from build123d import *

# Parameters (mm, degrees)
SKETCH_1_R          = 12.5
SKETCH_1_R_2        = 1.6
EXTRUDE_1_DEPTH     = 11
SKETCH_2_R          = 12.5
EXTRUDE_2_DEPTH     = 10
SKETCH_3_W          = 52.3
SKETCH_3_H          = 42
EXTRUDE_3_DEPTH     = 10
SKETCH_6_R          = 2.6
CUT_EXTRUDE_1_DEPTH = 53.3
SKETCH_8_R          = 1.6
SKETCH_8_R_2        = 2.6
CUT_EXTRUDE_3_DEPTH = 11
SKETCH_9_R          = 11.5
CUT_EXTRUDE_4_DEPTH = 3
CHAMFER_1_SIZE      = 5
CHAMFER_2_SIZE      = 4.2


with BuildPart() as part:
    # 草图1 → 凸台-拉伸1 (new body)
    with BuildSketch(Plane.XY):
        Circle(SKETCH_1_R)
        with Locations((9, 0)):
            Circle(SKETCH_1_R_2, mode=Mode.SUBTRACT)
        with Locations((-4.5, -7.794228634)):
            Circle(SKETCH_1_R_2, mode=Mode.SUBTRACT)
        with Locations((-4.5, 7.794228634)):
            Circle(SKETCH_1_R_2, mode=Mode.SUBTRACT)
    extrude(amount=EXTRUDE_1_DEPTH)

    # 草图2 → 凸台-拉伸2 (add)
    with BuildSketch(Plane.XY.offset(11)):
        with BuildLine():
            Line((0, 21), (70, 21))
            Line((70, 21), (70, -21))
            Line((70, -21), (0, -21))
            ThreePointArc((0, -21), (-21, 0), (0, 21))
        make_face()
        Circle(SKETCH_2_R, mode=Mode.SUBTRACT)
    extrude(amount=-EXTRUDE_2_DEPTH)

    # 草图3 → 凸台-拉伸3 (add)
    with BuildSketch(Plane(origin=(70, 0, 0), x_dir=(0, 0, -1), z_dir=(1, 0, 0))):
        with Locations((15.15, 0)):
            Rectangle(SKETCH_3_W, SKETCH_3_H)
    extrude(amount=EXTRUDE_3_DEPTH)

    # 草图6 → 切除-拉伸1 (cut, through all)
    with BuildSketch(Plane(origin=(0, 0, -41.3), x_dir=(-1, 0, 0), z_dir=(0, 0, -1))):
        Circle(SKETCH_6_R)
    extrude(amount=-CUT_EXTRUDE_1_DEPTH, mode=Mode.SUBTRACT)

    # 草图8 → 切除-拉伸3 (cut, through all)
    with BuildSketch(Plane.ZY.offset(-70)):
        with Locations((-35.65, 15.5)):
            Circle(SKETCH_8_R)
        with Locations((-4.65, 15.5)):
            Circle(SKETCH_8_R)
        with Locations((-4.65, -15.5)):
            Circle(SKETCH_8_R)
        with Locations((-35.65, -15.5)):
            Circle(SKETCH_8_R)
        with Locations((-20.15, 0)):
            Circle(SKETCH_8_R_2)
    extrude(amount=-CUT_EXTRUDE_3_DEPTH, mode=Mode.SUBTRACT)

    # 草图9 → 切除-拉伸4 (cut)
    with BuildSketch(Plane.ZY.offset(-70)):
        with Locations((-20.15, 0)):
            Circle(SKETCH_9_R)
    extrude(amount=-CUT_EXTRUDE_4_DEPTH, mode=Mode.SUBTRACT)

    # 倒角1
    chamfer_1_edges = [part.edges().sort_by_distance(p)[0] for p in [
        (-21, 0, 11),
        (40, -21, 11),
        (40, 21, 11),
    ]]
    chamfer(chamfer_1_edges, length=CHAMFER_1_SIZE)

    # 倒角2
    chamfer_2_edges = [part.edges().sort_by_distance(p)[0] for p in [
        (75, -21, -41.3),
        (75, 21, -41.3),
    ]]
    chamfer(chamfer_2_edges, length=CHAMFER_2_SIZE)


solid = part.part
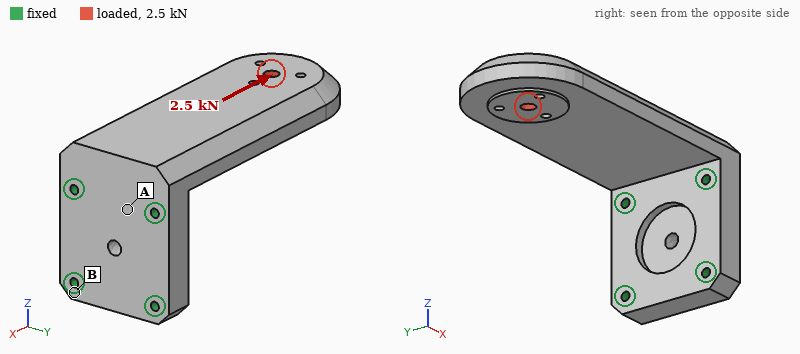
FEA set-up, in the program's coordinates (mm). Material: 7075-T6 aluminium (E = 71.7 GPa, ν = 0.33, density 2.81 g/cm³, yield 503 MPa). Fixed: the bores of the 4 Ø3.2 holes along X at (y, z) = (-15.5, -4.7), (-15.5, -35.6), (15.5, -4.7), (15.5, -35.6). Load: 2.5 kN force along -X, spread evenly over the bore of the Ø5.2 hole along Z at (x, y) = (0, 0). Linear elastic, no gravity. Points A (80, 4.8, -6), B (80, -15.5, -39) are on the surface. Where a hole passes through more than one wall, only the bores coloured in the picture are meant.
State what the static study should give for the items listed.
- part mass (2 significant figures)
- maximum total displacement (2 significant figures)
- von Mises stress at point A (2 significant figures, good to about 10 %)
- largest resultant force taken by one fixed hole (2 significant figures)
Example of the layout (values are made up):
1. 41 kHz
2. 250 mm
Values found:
1. 150 g
2. 76 µm
3. 13 MPa
4. 1.4 kN
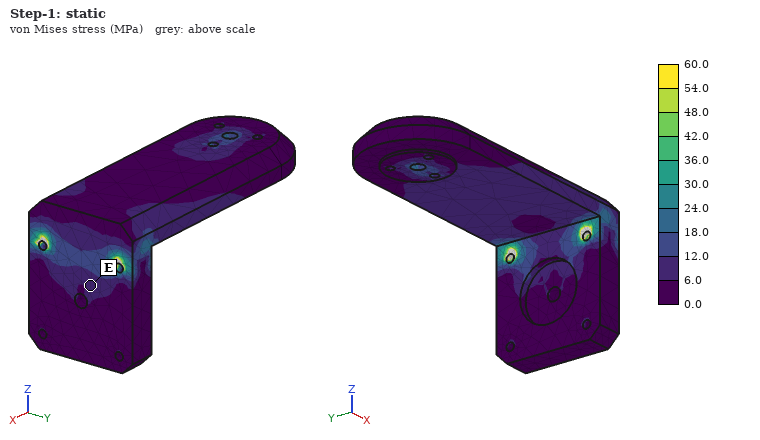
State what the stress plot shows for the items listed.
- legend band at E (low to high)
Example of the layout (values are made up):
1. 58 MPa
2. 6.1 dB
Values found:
1. 6.0 to 12.0 MPa
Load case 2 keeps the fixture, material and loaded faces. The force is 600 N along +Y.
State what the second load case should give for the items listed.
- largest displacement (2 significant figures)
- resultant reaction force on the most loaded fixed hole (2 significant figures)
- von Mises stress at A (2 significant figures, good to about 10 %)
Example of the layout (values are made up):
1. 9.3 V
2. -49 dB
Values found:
1. 73 µm
2. 1.4 kN
3. 7.6 MPa
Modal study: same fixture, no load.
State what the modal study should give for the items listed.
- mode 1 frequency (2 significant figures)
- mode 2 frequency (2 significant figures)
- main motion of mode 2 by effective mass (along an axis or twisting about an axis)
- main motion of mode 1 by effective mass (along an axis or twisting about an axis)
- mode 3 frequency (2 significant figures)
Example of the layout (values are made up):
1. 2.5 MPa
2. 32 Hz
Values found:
1. 820 Hz
2. 2400 Hz
3. along Y
4. along Z
5. 4400 Hz
